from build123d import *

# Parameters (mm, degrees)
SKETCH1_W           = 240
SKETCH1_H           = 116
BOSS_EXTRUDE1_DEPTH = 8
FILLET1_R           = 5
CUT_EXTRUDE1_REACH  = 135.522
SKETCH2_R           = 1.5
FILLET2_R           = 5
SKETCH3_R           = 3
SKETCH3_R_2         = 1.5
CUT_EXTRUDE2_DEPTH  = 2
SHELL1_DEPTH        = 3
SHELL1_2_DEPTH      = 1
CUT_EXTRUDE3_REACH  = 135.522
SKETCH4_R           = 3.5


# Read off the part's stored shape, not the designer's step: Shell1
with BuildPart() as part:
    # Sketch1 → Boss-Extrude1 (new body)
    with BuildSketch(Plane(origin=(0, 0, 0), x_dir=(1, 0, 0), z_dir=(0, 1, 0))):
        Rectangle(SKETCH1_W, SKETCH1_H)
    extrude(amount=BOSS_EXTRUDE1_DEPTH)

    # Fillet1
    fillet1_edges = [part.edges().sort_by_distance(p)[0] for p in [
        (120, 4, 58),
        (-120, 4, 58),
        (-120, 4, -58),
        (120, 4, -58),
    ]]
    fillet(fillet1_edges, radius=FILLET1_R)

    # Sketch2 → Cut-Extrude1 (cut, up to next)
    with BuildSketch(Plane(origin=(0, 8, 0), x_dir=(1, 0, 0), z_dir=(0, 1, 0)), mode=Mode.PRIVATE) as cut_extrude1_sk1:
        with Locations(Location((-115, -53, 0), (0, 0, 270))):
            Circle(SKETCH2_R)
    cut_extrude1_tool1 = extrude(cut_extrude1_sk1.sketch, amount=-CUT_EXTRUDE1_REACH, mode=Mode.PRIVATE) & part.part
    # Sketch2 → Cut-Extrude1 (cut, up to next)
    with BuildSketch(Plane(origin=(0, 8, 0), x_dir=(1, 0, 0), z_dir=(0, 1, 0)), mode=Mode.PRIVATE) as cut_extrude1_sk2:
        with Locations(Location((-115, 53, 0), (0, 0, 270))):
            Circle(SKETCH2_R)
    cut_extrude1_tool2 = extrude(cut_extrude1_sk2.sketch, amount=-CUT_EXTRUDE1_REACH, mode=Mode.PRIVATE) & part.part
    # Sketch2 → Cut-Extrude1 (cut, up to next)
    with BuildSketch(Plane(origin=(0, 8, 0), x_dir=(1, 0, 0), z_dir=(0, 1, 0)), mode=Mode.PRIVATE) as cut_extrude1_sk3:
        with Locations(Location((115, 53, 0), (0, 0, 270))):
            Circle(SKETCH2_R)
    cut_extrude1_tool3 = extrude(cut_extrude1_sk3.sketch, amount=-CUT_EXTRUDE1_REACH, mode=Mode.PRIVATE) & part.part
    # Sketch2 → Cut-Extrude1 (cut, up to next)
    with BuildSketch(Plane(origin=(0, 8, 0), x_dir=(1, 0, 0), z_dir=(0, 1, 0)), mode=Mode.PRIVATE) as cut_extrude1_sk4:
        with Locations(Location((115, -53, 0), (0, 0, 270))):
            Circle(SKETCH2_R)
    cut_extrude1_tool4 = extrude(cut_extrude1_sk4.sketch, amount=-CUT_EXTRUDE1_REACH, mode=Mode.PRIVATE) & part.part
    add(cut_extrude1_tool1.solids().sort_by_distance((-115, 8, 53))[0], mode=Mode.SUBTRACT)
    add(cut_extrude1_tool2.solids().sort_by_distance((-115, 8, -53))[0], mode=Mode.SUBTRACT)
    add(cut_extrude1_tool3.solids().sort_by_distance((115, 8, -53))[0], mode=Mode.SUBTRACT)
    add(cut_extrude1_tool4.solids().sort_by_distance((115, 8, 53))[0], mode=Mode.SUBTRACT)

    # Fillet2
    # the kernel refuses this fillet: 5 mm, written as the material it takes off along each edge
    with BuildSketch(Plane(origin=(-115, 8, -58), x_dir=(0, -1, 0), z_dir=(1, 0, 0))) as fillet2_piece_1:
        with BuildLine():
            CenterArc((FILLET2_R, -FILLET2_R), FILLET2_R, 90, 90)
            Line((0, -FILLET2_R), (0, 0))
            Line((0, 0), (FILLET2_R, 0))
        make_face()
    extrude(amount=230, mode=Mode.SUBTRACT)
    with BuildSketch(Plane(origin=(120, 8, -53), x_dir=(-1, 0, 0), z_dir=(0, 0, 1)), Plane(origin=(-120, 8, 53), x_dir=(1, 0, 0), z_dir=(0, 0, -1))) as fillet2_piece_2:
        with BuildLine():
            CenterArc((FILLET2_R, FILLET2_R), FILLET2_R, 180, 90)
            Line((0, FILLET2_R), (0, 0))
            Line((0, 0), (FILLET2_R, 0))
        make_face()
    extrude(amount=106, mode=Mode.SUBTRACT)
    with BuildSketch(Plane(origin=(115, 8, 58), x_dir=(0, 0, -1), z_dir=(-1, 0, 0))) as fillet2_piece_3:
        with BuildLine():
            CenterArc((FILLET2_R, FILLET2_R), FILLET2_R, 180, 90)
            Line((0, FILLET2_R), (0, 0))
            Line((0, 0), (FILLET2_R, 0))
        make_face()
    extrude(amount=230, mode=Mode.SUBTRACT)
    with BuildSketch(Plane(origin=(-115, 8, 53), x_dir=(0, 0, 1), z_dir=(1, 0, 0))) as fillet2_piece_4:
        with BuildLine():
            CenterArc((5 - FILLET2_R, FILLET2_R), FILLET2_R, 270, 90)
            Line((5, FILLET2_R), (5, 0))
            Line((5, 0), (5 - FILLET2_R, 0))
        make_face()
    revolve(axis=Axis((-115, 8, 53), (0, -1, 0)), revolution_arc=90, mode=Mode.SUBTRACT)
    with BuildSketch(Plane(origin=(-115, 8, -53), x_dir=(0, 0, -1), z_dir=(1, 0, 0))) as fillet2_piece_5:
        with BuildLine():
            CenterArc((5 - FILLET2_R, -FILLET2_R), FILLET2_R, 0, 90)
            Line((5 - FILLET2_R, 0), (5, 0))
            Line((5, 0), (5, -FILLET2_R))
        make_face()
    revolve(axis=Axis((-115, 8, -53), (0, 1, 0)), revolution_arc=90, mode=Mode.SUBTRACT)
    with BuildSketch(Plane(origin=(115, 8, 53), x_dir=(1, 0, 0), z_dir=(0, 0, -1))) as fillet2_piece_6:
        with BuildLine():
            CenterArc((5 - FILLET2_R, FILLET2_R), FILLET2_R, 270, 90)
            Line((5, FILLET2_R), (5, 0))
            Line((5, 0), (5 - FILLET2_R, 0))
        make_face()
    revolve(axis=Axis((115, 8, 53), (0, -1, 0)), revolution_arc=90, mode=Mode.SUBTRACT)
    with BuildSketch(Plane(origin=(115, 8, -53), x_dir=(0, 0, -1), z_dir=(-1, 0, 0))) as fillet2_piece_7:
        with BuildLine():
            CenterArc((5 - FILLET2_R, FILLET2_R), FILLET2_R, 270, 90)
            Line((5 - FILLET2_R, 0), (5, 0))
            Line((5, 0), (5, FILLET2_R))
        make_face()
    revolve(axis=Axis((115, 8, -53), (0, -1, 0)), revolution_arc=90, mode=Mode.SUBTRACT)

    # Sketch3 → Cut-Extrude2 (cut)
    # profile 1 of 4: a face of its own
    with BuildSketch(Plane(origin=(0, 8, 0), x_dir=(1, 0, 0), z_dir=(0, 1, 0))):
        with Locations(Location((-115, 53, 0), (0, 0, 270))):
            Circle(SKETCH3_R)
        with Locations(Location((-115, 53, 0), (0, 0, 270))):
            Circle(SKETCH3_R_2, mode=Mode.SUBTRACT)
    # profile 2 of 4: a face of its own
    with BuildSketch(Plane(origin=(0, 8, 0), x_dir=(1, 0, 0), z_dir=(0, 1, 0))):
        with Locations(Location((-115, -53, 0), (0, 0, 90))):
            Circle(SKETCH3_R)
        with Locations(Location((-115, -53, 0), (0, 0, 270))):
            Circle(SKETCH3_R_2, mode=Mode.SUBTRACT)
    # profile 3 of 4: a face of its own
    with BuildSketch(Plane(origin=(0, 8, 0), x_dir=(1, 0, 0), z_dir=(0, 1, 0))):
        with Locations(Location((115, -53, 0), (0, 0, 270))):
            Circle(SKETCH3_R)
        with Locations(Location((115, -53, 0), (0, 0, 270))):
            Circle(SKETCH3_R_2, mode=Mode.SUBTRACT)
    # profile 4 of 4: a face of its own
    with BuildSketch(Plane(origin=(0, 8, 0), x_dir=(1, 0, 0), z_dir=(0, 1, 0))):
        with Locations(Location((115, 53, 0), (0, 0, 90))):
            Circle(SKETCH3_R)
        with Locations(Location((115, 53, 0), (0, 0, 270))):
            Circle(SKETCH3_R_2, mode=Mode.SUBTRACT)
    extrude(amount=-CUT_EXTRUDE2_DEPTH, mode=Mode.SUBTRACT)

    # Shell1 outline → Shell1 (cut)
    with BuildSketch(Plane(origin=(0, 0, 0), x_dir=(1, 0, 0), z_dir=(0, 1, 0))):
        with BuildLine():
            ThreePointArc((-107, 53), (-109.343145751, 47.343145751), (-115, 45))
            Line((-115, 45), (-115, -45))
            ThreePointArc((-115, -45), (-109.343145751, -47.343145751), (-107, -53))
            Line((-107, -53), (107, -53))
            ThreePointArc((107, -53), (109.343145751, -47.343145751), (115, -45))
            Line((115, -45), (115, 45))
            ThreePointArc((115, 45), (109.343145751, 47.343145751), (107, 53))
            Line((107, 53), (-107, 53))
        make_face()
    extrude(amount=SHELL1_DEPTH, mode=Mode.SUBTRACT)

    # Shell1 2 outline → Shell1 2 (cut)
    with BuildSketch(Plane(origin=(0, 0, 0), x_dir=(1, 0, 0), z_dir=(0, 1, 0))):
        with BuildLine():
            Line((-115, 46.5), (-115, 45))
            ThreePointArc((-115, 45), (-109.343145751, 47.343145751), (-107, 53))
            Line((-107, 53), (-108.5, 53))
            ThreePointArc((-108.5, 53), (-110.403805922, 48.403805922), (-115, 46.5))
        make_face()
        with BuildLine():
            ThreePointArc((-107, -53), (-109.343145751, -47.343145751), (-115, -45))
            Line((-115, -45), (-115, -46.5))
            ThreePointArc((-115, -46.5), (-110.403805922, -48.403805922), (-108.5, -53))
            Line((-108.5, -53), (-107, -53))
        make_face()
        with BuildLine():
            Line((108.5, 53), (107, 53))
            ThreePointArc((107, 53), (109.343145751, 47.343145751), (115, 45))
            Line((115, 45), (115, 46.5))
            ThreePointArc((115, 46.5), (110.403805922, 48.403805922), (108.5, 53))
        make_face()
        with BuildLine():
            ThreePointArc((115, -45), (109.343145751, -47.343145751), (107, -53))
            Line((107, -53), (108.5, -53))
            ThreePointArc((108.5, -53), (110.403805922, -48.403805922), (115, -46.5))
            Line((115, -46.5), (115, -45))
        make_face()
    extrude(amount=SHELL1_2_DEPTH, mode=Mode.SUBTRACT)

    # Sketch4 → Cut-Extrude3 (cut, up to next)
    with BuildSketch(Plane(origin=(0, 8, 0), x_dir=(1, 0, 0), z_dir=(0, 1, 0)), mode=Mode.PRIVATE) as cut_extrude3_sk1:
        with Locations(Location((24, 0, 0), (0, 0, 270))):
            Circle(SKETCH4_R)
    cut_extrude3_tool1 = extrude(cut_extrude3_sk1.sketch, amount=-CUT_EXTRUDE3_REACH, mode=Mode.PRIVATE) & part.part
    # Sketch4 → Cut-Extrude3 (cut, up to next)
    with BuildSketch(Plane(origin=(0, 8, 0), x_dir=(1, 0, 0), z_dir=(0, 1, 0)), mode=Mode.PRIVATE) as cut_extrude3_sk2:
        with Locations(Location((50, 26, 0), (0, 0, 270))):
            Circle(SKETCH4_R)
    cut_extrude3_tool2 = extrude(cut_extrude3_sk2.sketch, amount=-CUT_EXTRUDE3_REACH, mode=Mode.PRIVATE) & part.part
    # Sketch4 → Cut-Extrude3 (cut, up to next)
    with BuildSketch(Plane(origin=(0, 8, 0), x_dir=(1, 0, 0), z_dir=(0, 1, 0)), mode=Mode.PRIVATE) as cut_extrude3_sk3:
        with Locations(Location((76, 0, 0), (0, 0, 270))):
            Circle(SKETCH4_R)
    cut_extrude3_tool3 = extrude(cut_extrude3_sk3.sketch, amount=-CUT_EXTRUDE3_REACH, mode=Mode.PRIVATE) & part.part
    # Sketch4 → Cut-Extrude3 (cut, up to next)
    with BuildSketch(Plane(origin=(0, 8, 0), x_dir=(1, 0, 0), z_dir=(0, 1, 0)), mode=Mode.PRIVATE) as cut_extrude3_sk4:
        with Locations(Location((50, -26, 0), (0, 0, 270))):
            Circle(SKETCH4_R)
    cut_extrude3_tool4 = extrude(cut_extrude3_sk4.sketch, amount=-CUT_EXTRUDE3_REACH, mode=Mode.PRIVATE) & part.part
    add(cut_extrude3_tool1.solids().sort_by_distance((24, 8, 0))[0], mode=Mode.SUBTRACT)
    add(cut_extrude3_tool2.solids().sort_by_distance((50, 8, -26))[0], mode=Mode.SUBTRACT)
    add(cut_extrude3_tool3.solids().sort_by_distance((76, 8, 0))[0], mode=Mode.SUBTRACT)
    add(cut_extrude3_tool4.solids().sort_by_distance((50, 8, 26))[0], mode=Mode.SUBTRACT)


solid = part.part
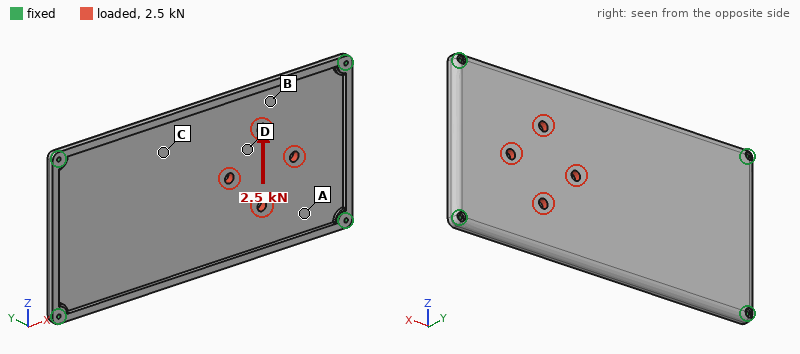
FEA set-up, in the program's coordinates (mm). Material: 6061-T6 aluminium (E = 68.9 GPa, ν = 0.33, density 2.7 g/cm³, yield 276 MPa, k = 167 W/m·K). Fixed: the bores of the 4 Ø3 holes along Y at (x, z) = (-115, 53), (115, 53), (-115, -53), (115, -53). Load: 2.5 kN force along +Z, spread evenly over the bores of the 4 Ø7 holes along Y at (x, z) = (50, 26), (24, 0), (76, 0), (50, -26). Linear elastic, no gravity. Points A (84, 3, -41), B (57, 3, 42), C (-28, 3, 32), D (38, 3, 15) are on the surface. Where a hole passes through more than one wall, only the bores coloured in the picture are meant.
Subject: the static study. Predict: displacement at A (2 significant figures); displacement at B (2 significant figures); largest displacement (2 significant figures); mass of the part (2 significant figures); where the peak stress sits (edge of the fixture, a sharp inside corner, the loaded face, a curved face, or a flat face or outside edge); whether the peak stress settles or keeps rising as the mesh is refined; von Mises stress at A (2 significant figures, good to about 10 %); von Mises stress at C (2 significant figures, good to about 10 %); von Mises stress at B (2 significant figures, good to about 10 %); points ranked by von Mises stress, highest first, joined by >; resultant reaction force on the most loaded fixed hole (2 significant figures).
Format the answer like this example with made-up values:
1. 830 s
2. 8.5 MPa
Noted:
1. 11 µm
2. 18 µm
3. 25 µm
4. 390 g
5. edge of the fixture
6. keeps rising
7. 6.6 MPa
8. 2.6 MPa
9. 4.3 MPa
10. A > B > C > D
11. 1.1 kN
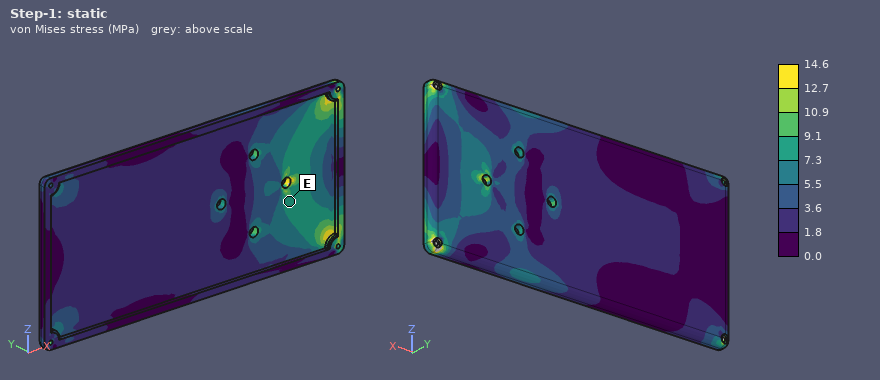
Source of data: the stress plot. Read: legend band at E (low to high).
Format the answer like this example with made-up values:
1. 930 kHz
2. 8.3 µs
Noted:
1. 7.3 to 9.1 MPa
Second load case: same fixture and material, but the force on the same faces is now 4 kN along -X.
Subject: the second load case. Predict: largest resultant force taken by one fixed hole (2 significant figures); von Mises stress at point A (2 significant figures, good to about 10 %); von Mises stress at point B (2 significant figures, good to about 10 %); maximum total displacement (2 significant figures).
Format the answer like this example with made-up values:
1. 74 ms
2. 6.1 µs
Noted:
1. 1.3 kN
2. 8.2 MPa
3. 4.8 MPa
4. 21 µm
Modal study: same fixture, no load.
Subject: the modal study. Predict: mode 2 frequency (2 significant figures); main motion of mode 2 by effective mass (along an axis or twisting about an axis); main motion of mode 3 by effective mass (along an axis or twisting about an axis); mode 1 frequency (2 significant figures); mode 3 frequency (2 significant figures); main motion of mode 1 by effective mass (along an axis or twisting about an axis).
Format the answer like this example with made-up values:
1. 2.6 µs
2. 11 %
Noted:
1. 840 Hz
2. twisting about X
3. twisting about Z
4. 460 Hz
5. 1300 Hz
6. along Y
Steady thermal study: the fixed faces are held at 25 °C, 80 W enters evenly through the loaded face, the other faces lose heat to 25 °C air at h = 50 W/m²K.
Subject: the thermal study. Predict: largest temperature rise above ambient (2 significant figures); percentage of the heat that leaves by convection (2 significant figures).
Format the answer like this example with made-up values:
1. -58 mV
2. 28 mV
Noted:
1. 33 K
2. 55 %
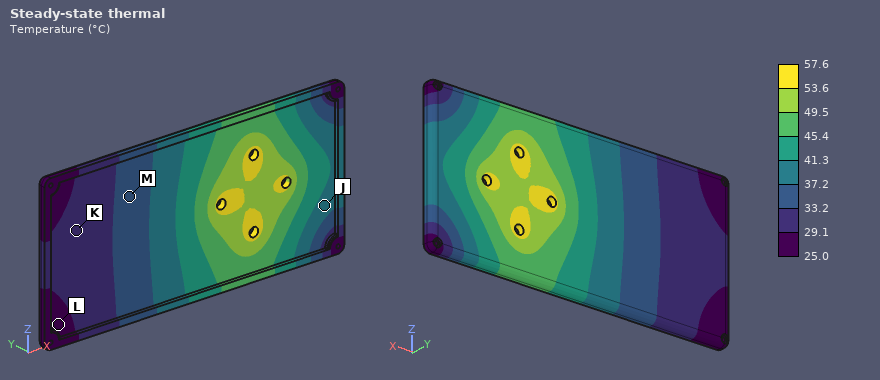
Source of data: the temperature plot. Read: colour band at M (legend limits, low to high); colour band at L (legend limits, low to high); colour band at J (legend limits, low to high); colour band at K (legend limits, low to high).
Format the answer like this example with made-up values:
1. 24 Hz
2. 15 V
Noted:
1. 33.2 to 37.2 °C
2. 25.0 to 29.1 °C
3. 37.2 to 41.3 °C
4. 29.1 to 33.2 °C
